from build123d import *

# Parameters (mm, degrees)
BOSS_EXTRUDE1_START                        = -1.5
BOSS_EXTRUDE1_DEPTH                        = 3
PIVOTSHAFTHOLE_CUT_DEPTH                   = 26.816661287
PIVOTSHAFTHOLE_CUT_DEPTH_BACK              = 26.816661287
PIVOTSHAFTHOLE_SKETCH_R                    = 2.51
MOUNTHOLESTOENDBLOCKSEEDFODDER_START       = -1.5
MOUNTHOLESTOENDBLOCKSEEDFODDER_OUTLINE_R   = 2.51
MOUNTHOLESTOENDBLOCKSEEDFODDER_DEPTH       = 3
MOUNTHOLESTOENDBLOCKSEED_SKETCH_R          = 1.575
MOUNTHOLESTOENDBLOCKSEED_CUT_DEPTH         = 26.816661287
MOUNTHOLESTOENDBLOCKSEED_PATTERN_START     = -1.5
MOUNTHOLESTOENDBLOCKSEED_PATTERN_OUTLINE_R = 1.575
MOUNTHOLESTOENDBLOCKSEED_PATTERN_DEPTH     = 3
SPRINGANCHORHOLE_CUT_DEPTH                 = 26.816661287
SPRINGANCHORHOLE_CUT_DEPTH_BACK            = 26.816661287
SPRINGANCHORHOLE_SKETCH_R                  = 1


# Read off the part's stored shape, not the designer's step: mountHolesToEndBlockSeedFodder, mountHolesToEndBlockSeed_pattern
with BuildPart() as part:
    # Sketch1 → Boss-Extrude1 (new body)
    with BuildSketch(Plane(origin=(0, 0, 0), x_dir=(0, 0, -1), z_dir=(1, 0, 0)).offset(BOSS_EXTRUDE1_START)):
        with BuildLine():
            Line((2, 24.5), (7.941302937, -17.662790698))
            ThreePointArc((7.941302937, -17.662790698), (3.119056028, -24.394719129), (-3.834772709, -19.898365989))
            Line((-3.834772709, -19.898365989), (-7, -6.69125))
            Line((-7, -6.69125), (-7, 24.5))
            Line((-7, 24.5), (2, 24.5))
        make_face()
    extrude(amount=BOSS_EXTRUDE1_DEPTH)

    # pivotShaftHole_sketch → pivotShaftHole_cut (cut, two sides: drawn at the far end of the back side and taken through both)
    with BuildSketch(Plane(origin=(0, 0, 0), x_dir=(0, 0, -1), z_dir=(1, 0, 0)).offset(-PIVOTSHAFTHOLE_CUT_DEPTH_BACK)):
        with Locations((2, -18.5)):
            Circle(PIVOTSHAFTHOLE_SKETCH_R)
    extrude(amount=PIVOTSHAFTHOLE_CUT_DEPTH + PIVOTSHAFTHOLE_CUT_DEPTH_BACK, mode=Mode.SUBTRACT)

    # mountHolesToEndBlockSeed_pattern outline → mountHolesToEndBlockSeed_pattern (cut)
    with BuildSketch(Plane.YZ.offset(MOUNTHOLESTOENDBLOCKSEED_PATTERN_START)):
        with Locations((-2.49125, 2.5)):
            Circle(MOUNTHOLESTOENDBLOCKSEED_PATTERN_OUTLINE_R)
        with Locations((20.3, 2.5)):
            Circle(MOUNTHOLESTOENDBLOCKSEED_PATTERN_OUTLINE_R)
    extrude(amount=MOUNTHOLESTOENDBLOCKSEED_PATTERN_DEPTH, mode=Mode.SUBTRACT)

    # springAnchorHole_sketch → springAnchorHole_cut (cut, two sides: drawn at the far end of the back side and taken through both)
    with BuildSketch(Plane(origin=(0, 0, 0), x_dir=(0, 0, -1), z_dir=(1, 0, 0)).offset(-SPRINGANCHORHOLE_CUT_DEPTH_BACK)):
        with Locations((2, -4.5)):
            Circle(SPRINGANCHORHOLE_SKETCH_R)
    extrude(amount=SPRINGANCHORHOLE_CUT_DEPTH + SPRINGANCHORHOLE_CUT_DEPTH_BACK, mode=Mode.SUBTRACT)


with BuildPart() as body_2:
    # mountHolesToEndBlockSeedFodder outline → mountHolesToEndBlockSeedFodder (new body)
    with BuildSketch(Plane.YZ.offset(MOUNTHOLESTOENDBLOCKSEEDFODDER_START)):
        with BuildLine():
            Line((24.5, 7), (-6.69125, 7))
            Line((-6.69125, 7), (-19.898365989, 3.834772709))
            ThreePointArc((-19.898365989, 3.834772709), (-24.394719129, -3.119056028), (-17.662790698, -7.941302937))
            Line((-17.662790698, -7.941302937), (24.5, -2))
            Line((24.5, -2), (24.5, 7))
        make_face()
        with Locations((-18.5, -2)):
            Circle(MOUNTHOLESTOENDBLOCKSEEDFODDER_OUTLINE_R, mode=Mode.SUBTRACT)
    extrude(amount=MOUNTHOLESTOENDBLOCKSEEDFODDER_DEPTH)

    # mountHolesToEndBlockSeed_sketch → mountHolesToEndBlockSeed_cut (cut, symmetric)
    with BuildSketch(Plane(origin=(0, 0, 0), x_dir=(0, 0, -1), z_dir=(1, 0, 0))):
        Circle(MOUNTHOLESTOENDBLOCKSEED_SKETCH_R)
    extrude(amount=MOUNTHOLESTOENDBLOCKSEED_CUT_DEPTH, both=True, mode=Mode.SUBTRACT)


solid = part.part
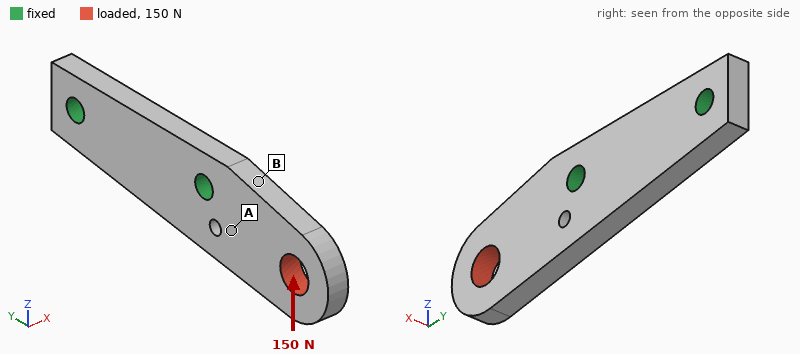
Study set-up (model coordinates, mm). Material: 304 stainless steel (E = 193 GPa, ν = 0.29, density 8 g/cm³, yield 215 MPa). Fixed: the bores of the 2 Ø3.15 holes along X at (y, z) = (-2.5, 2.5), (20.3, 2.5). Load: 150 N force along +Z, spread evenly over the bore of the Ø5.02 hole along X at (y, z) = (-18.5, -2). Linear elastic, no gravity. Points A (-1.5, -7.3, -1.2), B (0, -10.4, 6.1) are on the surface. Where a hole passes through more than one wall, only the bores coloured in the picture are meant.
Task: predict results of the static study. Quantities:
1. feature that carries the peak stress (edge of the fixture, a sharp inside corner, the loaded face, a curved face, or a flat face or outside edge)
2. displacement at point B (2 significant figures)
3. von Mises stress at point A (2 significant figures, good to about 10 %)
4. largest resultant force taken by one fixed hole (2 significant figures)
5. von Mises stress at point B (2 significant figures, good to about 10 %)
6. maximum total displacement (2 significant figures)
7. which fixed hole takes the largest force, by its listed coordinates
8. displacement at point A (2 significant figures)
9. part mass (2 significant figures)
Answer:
edge of the fixture
2.4 µm
6.9 MPa
220 N
17 MPa
7.6 µm
(-2.5, 2.5)
1.4 µm
12 g
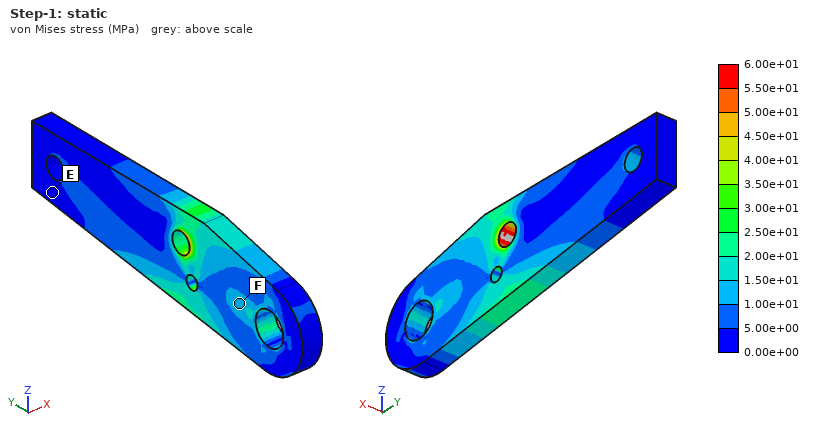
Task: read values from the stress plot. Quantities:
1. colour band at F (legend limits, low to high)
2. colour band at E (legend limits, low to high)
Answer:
1.00e+01 to 1.50e+01 MPa
0.00e+00 to 5.00e+00 MPa
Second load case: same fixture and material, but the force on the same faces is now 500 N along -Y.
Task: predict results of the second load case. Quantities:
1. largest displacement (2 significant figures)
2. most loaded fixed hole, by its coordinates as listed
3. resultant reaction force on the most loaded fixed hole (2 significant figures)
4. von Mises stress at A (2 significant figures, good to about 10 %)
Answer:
6.1 µm
(-2.5, 2.5)
410 N
17 MPa
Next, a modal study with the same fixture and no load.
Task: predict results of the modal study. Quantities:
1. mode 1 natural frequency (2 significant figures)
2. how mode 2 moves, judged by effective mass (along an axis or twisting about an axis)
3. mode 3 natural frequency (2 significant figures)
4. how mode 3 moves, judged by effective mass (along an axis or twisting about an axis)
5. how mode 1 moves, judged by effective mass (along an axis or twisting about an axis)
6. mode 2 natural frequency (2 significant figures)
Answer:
5700 Hz
along Z
17 kHz
twisting about Y
along X
15 kHz
